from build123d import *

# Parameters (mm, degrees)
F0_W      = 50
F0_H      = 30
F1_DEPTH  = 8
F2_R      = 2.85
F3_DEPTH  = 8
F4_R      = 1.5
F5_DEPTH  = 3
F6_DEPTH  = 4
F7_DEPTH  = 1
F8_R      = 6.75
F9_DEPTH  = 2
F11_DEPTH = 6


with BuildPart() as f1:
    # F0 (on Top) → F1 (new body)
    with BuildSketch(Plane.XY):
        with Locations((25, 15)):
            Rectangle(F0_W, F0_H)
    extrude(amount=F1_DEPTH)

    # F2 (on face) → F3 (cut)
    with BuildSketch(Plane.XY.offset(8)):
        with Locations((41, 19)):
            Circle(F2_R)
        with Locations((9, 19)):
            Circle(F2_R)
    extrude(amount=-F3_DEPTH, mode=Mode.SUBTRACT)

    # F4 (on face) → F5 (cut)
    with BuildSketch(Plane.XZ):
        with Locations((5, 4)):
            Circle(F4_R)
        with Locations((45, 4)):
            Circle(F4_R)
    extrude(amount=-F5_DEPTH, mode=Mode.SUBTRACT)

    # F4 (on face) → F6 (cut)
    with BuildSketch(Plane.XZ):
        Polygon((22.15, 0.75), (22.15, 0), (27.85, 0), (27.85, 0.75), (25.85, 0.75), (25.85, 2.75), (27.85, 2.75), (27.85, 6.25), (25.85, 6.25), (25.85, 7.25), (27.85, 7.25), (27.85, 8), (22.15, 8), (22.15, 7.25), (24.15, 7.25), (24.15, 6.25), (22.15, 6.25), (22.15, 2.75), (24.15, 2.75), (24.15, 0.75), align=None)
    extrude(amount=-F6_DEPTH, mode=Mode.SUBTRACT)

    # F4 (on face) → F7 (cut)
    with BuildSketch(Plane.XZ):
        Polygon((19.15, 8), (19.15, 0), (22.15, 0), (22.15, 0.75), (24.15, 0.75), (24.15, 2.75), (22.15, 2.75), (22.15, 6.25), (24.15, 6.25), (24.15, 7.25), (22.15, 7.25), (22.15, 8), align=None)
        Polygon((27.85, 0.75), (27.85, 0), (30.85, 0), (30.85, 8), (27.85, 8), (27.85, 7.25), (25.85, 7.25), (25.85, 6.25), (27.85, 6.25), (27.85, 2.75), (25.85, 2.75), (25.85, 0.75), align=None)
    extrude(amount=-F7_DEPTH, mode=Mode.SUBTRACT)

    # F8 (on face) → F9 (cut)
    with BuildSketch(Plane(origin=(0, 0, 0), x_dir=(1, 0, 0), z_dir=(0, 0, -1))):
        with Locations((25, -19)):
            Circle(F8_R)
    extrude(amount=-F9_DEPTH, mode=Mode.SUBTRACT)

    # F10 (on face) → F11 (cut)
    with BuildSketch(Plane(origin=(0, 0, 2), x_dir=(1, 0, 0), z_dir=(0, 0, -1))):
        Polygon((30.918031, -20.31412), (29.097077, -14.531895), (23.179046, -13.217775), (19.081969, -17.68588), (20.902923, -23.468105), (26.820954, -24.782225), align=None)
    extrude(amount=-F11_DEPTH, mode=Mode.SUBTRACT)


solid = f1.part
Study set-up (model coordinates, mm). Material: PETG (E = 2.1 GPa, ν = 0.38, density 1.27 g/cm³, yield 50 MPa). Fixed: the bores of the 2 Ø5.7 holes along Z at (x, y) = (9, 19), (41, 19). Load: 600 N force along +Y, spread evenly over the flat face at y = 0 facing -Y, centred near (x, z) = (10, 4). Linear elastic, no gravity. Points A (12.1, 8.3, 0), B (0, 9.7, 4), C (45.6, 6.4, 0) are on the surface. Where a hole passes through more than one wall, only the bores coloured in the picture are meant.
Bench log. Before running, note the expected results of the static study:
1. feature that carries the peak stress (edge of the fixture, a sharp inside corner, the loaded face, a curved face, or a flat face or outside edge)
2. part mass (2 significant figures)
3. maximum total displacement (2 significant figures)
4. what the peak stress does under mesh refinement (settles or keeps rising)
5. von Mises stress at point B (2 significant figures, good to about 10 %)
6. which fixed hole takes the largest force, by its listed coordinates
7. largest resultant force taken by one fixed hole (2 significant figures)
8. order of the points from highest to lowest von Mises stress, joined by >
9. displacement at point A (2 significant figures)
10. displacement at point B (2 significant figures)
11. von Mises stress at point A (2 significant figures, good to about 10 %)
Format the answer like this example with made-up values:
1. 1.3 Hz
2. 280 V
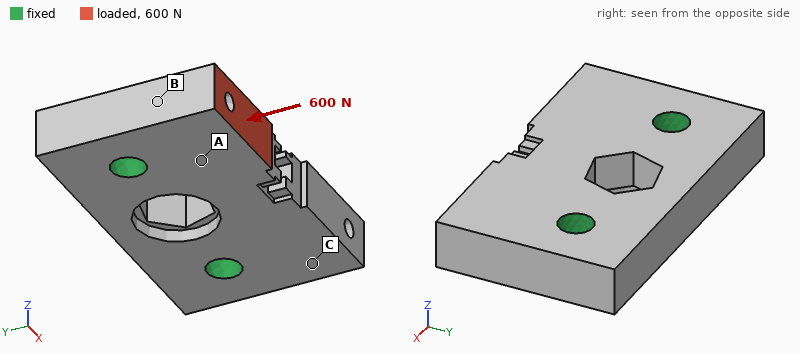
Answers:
1. edge of the fixture
2. 13 g
3. 49 µm
4. keeps rising
5. 3.3 MPa
6. (9, 19)
7. 570 N
8. A > B > C
9. 20 µm
10. 29 µm
11. 4.5 MPa
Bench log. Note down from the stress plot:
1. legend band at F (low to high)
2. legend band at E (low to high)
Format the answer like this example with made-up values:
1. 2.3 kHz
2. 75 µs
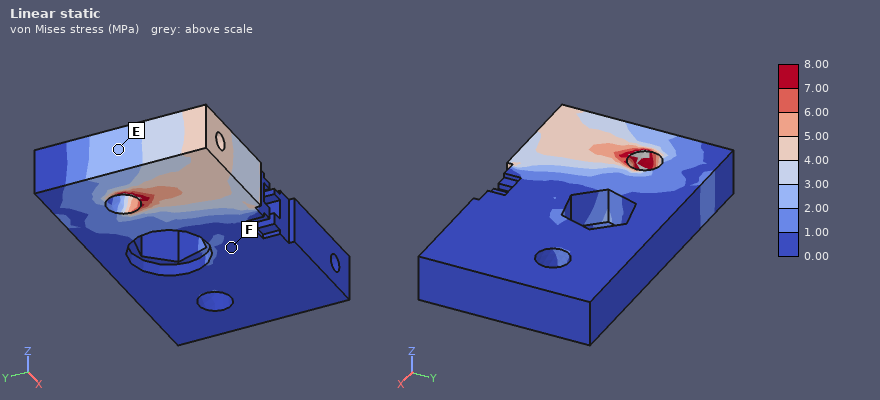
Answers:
1. 0.00 to 1.00 MPa
2. 2.00 to 3.00 MPa
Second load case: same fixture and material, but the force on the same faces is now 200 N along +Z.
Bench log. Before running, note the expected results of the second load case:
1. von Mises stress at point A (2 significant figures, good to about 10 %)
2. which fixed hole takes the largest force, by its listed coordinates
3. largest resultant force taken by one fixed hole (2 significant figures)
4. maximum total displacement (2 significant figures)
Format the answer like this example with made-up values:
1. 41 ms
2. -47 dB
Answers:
1. 6.5 MPa
2. (9, 19)
3. 190 N
4. 0.25 mm
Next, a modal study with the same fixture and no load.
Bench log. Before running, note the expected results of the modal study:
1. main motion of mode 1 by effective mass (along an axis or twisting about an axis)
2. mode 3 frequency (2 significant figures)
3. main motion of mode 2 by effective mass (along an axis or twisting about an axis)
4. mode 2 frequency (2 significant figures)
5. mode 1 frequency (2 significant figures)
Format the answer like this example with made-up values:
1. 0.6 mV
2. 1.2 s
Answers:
1. along Z
2. 6900 Hz
3. twisting about Y
4. 5200 Hz
5. 3900 Hz
